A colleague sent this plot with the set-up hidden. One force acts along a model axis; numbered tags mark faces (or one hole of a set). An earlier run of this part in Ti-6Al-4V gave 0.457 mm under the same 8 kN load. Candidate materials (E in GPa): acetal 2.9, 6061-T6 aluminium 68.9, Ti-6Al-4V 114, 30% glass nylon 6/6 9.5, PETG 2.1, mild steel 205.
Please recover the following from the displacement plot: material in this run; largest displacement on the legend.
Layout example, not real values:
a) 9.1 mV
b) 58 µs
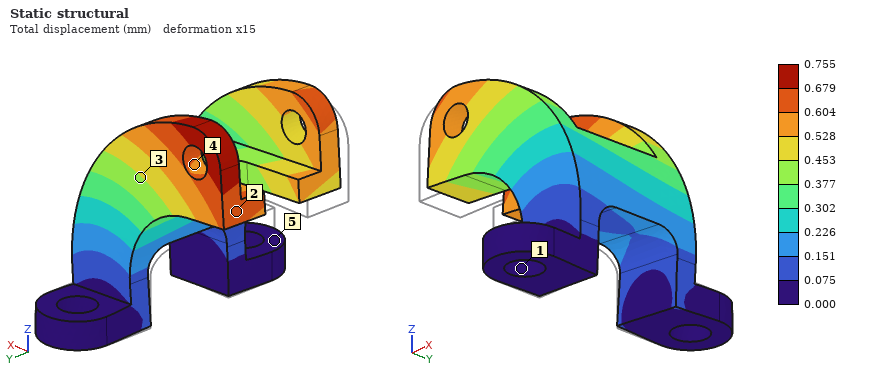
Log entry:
a) 6061-T6 aluminium
b) 0.755 mm
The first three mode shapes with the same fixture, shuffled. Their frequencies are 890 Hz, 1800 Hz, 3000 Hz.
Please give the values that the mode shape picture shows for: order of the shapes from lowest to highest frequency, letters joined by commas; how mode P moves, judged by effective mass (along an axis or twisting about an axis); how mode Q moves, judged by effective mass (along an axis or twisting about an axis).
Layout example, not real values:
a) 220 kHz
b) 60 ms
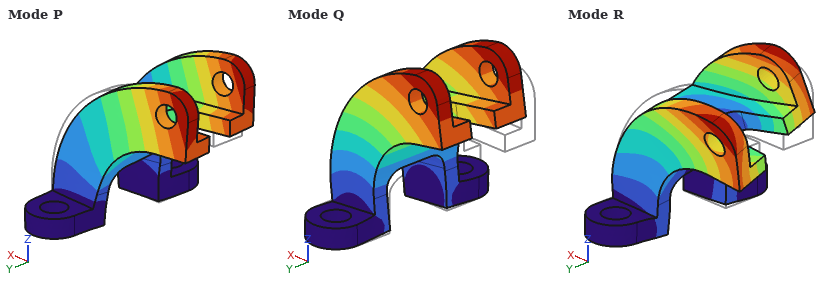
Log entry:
a) Q, P, R
b) along Y
c) along X
